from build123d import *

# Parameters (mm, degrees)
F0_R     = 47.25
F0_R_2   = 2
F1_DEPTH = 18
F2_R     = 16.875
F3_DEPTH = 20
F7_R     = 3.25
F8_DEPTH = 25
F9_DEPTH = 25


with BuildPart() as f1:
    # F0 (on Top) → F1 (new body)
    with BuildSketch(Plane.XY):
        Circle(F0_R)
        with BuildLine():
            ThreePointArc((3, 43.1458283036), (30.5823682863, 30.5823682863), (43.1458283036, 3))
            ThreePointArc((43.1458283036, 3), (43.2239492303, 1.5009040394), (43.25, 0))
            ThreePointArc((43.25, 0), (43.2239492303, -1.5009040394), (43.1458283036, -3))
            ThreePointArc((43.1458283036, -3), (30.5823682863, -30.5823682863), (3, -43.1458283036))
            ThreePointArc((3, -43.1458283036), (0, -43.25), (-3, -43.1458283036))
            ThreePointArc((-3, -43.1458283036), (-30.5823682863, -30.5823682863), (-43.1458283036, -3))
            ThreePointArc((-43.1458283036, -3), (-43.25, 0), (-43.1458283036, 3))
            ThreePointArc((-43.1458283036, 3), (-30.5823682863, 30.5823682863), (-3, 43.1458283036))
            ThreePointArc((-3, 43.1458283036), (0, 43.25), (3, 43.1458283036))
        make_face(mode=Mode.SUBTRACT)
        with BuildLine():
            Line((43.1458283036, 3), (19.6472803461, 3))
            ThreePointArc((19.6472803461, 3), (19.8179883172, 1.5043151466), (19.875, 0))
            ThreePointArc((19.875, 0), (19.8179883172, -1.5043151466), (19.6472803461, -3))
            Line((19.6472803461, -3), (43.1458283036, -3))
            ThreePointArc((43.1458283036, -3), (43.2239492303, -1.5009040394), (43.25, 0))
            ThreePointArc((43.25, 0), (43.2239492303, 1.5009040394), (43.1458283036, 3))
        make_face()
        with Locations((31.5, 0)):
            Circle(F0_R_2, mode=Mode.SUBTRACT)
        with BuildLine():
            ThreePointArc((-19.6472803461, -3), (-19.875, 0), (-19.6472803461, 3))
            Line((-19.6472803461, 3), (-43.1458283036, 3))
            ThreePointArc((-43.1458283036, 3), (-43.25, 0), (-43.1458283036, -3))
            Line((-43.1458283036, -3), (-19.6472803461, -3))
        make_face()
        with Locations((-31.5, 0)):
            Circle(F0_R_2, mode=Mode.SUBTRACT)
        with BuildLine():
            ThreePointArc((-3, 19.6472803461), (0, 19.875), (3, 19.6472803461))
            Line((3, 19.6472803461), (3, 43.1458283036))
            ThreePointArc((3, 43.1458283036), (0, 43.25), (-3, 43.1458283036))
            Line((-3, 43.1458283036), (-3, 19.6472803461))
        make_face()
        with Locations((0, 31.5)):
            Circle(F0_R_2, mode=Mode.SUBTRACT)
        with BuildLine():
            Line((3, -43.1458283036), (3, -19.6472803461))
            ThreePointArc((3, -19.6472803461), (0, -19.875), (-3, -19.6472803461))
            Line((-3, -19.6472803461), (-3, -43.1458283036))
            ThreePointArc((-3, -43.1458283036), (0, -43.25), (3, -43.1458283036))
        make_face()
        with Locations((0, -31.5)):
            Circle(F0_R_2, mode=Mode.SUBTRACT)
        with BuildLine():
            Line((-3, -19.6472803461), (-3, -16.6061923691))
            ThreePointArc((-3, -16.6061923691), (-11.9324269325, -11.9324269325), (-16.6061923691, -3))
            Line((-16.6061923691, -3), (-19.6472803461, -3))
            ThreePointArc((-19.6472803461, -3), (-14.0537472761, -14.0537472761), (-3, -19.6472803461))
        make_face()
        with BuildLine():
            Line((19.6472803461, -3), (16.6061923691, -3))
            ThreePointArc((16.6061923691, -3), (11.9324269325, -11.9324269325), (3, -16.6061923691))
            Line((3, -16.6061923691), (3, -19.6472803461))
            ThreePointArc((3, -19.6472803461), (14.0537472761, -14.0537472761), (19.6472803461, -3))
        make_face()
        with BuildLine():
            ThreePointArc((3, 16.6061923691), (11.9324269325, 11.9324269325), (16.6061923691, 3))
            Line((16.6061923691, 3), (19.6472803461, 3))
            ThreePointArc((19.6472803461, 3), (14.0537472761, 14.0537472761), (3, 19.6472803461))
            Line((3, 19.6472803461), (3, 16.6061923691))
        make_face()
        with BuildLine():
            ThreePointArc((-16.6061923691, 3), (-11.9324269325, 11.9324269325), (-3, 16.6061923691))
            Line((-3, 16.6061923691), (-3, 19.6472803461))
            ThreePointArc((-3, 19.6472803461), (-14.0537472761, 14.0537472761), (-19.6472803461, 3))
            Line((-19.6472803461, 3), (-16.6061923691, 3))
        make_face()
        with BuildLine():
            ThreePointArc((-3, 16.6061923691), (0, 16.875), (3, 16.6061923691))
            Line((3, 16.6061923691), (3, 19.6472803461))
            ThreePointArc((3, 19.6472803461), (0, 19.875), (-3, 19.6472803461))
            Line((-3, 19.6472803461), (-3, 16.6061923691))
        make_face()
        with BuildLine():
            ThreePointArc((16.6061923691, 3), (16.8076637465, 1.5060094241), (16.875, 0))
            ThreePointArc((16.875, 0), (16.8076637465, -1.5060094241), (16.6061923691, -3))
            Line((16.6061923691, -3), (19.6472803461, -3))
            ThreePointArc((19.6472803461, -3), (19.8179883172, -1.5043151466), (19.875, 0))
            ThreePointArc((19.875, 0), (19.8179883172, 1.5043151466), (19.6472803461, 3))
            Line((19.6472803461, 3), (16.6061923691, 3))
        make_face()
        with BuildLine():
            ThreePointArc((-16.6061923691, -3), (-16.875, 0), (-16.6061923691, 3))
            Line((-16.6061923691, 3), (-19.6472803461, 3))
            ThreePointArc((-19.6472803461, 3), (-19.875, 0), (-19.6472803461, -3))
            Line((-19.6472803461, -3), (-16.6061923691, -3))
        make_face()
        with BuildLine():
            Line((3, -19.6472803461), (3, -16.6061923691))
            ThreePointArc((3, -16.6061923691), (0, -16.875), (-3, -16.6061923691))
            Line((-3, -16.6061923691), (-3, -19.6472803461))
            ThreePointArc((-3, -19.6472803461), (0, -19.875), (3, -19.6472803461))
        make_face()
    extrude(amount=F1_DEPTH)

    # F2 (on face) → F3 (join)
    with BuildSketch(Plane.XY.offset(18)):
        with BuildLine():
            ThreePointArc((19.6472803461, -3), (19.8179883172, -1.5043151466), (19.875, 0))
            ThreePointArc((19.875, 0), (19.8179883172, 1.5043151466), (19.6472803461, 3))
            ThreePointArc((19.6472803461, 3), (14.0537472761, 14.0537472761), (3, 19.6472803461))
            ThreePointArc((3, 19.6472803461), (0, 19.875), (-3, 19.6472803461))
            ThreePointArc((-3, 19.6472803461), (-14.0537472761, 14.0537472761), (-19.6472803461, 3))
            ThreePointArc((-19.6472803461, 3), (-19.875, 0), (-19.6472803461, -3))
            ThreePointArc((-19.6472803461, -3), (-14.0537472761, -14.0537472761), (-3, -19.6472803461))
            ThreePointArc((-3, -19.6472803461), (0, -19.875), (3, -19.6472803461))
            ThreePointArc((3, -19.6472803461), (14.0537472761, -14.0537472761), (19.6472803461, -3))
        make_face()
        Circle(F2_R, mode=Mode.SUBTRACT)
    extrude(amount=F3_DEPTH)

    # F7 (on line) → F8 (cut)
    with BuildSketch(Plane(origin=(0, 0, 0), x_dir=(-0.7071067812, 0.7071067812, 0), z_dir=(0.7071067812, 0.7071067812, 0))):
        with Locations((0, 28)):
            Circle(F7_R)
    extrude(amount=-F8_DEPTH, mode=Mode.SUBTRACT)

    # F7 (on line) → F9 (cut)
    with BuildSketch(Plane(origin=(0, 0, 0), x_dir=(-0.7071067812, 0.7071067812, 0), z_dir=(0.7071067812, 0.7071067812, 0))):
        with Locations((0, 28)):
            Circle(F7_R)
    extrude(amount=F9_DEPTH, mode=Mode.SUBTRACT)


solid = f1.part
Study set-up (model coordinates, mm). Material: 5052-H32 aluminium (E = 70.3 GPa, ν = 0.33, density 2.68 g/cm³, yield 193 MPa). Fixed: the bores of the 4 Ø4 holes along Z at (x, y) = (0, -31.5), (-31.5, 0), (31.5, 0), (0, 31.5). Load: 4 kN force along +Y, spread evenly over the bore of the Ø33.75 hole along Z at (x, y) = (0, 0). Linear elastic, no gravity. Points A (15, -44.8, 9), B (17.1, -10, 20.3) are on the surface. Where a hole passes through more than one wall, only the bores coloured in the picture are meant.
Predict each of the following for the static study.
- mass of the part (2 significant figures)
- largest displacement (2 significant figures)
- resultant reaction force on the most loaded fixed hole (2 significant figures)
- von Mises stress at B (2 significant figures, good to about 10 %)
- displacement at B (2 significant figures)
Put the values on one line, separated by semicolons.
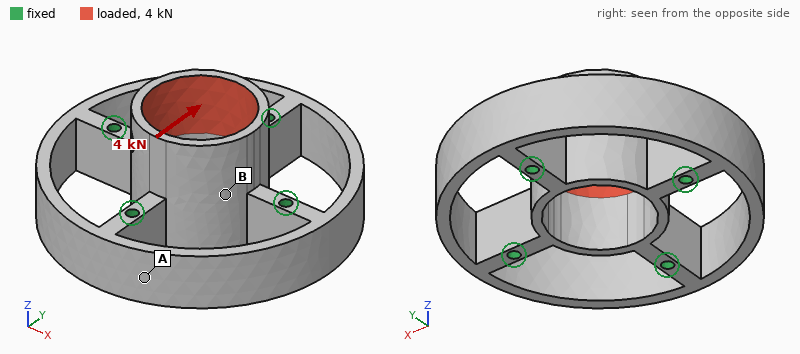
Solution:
110 g; 48 µm; 1.9 kN; 31 MPa; 33 µm
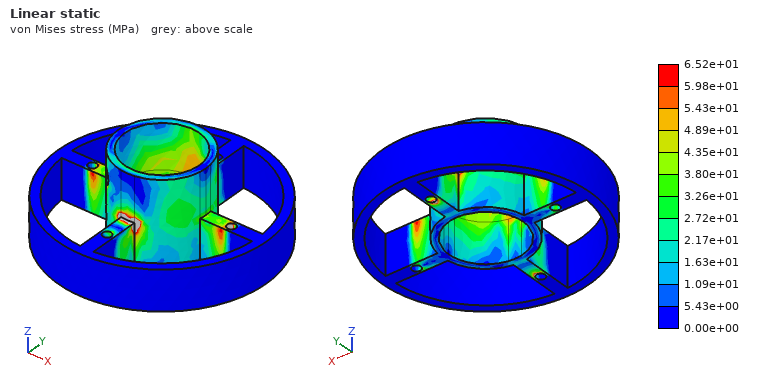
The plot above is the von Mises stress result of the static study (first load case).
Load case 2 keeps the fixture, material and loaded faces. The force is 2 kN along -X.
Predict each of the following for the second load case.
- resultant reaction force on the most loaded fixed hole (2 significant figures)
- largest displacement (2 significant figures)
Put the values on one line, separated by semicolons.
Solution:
970 N; 24 µm
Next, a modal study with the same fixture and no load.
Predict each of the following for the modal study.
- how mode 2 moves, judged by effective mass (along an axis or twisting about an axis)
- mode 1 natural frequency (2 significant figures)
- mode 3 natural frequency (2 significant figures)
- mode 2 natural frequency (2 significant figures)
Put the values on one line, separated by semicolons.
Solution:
twisting about Z; 5400 Hz; 6700 Hz; 5900 Hz
